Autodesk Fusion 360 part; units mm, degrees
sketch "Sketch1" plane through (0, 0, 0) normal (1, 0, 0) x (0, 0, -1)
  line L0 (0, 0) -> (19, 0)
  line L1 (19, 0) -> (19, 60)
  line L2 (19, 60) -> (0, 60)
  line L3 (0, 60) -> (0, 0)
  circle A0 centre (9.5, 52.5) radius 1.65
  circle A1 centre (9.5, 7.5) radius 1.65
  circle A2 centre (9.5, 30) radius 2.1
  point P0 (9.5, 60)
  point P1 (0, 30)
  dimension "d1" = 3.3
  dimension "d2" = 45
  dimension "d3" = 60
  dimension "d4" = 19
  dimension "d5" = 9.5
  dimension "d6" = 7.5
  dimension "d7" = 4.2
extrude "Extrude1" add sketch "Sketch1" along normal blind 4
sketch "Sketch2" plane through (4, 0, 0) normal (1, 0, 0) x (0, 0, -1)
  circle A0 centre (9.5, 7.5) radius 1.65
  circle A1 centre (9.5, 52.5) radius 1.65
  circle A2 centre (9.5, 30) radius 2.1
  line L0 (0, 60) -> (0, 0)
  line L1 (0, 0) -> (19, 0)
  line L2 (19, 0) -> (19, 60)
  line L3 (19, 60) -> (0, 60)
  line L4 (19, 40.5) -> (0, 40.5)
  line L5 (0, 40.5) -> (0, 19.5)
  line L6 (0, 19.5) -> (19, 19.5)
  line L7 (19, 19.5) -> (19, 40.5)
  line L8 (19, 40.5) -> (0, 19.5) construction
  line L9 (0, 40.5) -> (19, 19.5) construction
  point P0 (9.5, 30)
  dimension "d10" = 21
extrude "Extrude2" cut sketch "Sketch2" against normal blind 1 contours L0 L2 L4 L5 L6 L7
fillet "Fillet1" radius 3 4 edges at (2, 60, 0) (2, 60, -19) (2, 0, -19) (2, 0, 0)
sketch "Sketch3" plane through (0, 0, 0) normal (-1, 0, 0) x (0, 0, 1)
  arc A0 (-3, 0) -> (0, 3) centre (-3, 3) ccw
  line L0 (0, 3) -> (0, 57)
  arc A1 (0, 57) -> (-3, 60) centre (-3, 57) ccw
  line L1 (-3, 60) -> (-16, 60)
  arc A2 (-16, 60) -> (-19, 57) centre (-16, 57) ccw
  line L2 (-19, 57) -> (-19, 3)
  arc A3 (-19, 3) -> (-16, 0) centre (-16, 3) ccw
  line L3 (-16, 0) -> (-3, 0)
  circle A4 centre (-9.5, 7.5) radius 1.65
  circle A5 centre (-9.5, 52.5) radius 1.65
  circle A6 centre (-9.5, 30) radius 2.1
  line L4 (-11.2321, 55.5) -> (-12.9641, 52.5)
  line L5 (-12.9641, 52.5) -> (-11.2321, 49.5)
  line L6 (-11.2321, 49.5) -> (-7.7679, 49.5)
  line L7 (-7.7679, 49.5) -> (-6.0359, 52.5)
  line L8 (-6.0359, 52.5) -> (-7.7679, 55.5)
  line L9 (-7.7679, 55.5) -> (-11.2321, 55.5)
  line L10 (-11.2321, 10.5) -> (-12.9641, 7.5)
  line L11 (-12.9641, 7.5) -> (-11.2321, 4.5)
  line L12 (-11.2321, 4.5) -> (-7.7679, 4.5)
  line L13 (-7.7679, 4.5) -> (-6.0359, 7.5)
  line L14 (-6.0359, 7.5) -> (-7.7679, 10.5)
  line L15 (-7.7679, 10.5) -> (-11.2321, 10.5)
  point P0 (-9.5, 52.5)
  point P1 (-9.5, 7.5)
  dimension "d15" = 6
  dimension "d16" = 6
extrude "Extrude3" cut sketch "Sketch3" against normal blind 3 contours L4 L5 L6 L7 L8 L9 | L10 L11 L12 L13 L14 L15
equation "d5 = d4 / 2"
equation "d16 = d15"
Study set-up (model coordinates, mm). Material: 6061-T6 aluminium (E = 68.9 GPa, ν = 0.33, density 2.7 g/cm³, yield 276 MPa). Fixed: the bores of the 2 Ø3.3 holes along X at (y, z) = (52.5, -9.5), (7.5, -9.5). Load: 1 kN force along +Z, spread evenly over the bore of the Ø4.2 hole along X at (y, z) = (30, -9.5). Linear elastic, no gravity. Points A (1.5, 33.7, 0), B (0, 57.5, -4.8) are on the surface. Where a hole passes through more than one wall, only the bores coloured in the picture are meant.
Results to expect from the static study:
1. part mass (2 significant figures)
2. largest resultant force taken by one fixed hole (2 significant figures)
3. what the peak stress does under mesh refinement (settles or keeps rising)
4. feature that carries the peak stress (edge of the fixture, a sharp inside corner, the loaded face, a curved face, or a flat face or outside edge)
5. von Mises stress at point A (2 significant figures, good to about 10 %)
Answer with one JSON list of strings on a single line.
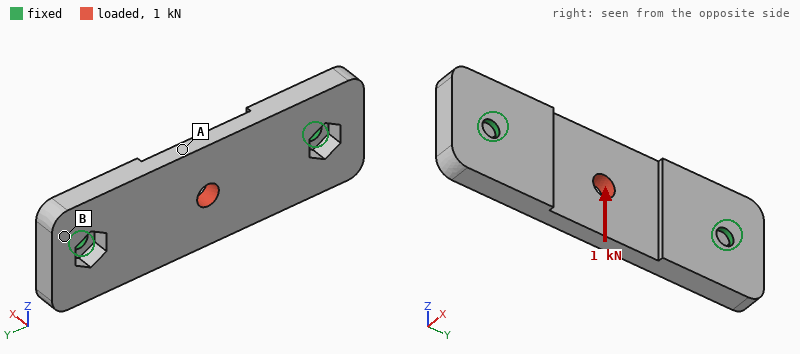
["10 g", "500 N", "keeps rising", "edge of the fixture", "52 MPa"]
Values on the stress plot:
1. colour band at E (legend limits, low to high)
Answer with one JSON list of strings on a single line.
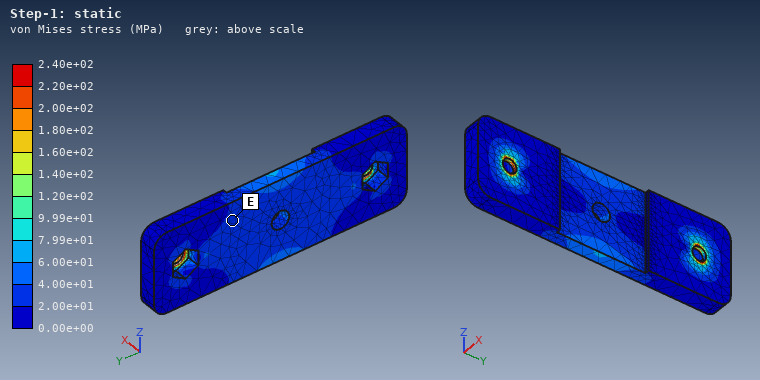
["2.00e+01 to 4.00e+01 MPa"]
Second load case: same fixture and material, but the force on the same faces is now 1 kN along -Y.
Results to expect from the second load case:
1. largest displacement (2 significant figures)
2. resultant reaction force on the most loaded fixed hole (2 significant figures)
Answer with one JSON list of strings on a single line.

["7.5 µm", "500 N"]
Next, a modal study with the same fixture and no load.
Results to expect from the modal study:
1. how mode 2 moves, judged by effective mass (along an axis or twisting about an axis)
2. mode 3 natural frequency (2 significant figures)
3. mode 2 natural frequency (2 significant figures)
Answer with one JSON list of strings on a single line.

["along X", "11 kHz", "6600 Hz"]
